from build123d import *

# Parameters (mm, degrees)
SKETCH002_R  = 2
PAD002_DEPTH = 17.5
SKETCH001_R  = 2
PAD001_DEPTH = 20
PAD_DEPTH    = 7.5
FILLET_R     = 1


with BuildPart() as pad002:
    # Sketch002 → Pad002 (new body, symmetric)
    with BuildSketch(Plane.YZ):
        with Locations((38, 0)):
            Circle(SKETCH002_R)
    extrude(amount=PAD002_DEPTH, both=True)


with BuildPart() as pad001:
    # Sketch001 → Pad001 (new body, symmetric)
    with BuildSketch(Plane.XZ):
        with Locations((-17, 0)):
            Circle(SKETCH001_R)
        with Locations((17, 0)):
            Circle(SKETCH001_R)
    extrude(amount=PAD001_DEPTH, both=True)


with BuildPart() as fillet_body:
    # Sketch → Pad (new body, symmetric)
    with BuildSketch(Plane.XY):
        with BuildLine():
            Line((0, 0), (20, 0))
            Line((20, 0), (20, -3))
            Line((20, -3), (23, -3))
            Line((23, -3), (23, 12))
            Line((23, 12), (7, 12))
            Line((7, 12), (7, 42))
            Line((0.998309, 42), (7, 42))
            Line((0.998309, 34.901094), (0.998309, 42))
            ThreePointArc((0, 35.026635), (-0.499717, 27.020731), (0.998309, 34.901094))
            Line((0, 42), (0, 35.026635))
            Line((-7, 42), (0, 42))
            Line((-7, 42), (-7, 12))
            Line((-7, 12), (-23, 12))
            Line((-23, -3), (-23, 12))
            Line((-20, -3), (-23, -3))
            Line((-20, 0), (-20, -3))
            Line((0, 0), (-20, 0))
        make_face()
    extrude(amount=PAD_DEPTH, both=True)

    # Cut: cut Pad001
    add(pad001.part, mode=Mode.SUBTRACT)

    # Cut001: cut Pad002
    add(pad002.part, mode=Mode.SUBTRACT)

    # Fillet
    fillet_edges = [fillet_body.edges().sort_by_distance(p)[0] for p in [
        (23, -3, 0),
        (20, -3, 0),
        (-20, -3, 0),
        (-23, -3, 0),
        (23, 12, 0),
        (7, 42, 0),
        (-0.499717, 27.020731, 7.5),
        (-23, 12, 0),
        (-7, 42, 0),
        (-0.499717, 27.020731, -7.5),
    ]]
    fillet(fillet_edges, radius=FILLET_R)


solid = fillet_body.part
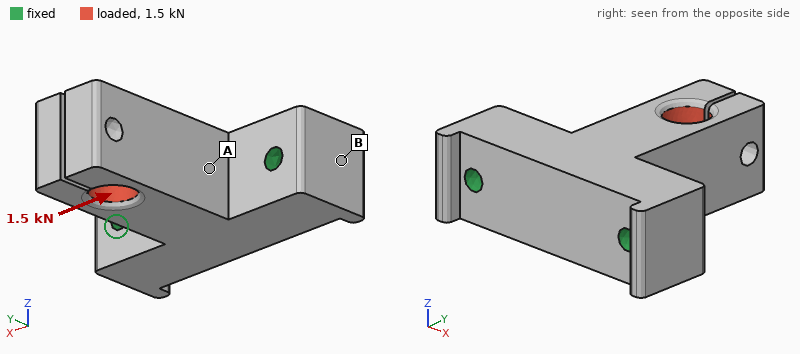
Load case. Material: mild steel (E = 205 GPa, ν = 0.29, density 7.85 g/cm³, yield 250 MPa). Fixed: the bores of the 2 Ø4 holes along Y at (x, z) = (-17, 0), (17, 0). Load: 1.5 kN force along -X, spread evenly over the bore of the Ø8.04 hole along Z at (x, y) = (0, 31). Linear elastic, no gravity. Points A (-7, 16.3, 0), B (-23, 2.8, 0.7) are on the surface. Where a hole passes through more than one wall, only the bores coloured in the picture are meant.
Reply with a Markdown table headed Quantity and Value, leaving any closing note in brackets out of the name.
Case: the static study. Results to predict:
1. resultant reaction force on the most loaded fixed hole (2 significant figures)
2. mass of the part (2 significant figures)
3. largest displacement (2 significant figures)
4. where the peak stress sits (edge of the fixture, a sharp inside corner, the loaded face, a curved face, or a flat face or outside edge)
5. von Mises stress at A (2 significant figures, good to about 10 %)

| Quantity | Value |
|---|---|
| resultant reaction force on the most loaded fixed hole | 1.5 kN |
| mass of the part | 110 g |
| largest displacement | 35 µm |
| where the peak stress sits | the loaded face |
| von Mises stress at A | 47 MPa |
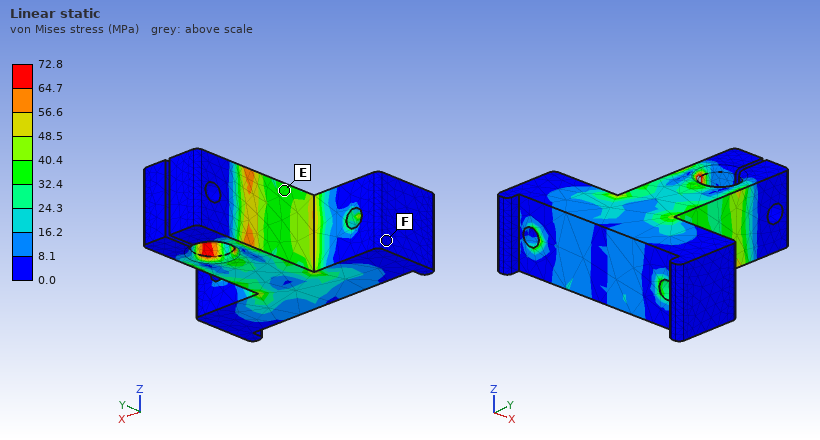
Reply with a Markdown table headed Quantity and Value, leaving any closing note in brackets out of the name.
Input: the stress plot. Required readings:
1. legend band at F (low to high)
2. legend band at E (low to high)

| Quantity | Value |
|---|---|
| legend band at F | 0.0 to 8.1 MPa |
| legend band at E | 32.4 to 40.4 MPa |
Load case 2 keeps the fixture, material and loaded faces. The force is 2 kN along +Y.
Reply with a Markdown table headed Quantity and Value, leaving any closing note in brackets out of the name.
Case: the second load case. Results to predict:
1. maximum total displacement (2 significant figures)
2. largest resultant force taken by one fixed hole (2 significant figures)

| Quantity | Value |
|---|---|
| maximum total displacement | 18 µm |
| largest resultant force taken by one fixed hole | 1.0 kN |
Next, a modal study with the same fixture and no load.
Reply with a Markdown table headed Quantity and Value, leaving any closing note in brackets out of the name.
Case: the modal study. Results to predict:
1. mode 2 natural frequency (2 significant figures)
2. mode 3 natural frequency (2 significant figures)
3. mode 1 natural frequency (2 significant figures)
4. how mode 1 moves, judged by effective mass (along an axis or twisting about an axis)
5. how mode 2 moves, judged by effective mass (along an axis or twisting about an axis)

| Quantity | Value |
|---|---|
| mode 2 natural frequency | 6800 Hz |
| mode 3 natural frequency | 8300 Hz |
| mode 1 natural frequency | 6500 Hz |
| how mode 1 moves, judged by effective mass | along Z |
| how mode 2 moves, judged by effective mass | along X |
